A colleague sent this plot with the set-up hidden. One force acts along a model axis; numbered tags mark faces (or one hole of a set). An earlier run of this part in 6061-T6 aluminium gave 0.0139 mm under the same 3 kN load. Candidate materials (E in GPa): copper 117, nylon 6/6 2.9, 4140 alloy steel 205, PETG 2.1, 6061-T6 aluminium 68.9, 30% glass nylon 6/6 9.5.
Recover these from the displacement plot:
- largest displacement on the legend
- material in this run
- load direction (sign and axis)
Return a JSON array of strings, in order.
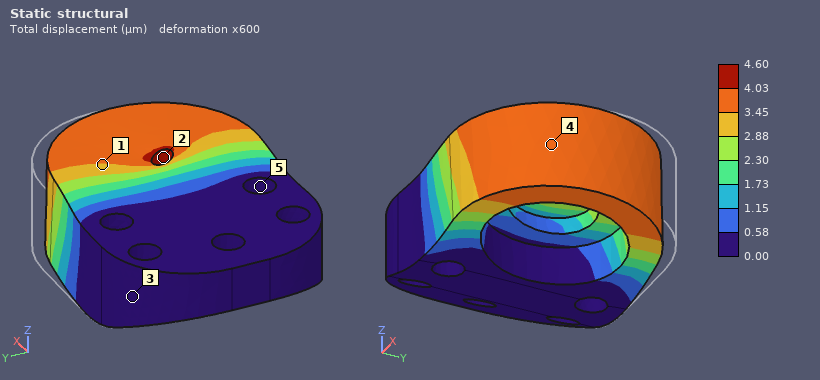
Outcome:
["4.60 µm", "4140 alloy steel", "-Y"]
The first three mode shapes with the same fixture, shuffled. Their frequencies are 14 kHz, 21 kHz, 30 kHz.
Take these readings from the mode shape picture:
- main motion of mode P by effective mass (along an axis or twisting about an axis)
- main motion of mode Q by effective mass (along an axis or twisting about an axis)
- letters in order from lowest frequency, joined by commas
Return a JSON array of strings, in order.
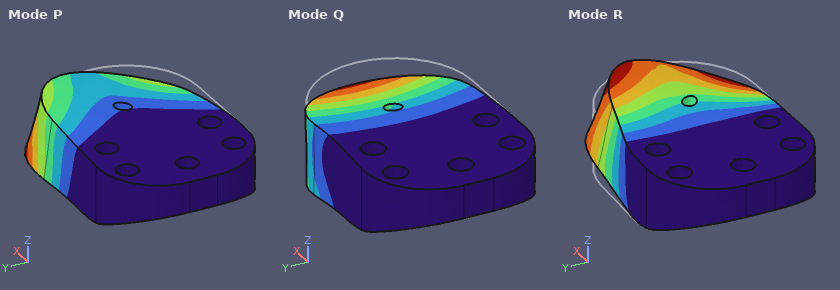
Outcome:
["along Y", "along Z", "Q, P, R"]
